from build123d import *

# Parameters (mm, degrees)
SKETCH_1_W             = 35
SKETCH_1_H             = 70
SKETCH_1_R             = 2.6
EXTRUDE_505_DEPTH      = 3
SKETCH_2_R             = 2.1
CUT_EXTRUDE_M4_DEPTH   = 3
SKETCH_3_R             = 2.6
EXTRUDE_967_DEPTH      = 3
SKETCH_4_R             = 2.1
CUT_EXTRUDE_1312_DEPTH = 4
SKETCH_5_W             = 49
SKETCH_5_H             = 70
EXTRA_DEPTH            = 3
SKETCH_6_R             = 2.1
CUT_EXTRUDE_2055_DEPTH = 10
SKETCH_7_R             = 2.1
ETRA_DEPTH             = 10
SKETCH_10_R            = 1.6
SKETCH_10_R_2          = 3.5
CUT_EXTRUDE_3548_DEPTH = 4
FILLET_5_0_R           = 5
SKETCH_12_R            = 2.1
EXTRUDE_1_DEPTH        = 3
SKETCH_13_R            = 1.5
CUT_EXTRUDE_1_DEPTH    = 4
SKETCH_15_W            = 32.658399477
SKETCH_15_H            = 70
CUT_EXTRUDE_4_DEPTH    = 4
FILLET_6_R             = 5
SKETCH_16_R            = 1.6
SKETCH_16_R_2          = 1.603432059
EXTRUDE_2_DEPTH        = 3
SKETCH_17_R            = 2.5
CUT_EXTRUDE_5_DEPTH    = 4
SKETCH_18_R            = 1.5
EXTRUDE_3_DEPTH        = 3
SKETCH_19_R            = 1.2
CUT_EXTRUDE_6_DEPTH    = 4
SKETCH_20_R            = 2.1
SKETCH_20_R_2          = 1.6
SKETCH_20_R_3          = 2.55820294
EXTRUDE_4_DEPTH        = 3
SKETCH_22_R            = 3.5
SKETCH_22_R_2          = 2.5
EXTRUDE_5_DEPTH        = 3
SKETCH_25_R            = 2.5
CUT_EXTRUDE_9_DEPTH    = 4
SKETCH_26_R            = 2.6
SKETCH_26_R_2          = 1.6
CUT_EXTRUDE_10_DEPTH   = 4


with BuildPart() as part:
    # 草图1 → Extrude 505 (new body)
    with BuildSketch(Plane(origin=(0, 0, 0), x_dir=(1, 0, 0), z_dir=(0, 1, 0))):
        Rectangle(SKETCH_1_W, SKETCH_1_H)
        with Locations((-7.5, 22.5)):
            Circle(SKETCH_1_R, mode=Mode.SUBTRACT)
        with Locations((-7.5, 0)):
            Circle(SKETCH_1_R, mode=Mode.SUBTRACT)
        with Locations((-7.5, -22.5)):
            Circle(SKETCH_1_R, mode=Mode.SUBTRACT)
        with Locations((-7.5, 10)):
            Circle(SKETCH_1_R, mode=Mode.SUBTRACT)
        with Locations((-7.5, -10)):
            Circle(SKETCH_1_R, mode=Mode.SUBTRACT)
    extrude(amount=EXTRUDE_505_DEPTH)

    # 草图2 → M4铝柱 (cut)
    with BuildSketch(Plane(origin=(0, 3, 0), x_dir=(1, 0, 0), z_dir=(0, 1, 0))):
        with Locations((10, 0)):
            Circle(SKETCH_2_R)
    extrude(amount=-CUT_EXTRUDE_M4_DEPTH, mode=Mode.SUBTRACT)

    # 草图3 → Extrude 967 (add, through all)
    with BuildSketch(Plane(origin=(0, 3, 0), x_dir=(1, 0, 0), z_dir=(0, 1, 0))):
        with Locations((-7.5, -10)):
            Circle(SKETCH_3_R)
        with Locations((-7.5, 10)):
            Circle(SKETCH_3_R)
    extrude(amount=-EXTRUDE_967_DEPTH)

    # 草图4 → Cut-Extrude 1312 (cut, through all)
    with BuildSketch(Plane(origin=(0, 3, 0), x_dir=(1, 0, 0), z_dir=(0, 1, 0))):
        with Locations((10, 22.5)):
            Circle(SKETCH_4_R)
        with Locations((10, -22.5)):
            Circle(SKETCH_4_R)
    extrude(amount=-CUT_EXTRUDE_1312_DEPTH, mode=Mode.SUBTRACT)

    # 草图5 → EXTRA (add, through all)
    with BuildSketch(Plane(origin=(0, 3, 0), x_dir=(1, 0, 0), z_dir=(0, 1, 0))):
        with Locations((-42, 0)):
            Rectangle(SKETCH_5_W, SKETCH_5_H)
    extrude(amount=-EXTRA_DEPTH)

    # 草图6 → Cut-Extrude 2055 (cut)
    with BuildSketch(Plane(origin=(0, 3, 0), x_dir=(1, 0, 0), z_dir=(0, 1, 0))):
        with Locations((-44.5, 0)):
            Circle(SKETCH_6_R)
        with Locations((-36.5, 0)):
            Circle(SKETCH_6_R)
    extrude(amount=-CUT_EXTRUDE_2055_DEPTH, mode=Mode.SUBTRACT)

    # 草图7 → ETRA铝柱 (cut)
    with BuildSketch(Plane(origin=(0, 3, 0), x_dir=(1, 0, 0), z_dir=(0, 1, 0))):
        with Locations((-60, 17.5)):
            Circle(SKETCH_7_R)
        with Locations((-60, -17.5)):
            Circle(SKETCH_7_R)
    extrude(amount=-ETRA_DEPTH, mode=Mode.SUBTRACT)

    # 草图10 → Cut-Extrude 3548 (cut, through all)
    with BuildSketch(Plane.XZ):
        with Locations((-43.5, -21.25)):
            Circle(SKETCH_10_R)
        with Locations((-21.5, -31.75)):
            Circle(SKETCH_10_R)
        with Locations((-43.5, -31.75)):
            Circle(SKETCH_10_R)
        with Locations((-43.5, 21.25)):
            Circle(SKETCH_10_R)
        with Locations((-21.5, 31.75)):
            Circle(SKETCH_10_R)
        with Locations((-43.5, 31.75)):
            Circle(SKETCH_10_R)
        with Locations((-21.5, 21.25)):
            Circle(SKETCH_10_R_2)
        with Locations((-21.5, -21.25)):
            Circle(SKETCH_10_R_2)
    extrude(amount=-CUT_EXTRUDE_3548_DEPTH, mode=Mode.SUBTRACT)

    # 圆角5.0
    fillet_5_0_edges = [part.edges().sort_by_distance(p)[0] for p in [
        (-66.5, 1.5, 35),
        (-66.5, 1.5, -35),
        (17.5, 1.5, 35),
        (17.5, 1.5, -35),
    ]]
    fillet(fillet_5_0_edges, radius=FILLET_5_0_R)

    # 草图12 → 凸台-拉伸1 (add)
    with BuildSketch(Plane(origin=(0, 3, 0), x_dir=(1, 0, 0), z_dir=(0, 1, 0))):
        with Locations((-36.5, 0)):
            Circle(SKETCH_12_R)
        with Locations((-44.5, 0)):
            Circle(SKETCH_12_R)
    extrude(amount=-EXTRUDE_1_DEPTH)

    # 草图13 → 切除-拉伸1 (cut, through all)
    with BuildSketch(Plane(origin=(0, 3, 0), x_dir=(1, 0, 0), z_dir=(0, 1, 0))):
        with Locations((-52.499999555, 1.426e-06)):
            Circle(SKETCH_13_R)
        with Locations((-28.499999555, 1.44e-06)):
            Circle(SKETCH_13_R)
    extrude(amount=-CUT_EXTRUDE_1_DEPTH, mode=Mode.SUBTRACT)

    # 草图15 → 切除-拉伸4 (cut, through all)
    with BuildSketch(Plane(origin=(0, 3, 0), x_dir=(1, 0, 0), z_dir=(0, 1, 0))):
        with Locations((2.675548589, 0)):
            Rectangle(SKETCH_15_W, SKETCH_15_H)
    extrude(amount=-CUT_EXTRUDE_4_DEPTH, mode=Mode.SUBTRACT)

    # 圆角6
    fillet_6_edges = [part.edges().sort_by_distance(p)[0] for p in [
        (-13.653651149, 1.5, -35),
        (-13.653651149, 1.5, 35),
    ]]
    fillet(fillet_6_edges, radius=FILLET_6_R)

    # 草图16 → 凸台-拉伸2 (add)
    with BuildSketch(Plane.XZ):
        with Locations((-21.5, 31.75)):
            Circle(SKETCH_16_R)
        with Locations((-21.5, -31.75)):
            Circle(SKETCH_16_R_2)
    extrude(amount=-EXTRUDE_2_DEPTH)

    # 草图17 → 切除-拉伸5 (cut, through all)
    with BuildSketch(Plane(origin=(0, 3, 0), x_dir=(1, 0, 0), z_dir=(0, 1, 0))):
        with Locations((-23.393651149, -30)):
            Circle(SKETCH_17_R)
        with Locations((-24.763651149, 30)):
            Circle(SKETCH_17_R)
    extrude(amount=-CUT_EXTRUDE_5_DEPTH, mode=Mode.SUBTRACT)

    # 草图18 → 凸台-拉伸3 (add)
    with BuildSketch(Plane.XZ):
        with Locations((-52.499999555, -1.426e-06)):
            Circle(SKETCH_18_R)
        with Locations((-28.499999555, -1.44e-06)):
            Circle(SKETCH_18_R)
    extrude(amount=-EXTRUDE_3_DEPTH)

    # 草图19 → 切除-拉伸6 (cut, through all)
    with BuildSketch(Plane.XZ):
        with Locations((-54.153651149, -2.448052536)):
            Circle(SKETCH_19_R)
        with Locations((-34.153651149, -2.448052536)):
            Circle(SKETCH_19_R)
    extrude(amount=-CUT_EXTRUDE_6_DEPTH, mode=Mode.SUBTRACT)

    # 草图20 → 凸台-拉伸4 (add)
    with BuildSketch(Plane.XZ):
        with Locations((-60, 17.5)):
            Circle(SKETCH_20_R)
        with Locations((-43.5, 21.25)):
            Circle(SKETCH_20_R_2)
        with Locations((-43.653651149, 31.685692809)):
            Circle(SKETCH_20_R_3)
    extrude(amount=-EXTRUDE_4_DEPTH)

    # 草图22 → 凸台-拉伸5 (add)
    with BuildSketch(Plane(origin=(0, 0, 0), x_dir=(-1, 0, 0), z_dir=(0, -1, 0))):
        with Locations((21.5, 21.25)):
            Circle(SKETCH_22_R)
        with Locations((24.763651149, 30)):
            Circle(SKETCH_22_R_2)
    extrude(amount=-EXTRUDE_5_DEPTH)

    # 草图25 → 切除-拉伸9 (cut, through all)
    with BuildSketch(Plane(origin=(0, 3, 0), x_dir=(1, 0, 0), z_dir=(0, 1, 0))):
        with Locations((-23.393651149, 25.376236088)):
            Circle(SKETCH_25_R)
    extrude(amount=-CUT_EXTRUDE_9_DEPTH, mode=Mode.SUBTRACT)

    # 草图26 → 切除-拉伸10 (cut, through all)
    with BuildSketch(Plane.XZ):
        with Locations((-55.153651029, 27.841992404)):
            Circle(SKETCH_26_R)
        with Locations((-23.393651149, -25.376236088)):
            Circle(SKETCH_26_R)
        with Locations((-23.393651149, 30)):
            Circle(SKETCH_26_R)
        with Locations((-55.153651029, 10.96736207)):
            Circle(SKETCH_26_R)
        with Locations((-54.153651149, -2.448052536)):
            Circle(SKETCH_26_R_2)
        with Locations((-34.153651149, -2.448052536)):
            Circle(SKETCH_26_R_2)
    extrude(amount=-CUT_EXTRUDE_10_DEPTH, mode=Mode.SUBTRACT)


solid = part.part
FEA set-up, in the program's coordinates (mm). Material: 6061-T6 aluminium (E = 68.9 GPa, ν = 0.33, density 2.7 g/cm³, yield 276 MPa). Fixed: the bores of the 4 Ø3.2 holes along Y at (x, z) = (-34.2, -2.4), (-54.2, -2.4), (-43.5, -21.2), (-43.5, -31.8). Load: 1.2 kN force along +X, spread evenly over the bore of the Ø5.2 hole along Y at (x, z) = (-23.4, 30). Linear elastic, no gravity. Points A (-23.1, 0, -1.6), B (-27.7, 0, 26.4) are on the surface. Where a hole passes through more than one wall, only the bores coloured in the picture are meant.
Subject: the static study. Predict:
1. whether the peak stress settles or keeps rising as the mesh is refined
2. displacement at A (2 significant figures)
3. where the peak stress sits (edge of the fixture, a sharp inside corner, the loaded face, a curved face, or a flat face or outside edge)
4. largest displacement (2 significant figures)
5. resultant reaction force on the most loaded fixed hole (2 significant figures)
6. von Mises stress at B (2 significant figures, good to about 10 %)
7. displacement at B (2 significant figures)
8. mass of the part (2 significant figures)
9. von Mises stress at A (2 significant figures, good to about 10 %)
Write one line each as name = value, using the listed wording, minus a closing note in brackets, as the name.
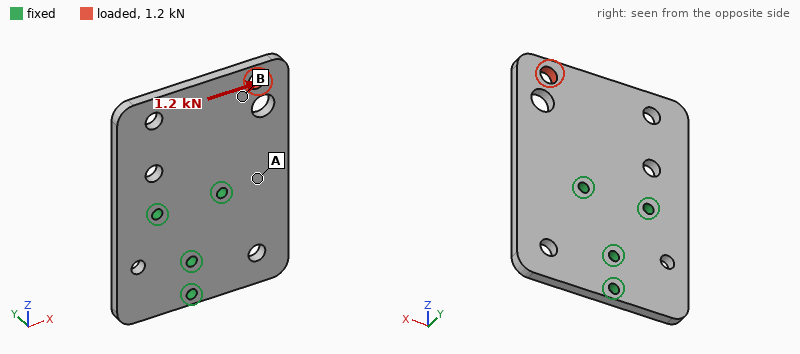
whether the peak stress settles or keeps rising as the mesh is refined = keeps rising
displacement at A = 7.9 µm
where the peak stress sits = edge of the fixture
largest displacement = 43 µm
resultant reaction force on the most loaded fixed hole = 1.4 kN
von Mises stress at B = 32 MPa
displacement at B = 29 µm
mass of the part = 28 g
von Mises stress at A = 15 MPa
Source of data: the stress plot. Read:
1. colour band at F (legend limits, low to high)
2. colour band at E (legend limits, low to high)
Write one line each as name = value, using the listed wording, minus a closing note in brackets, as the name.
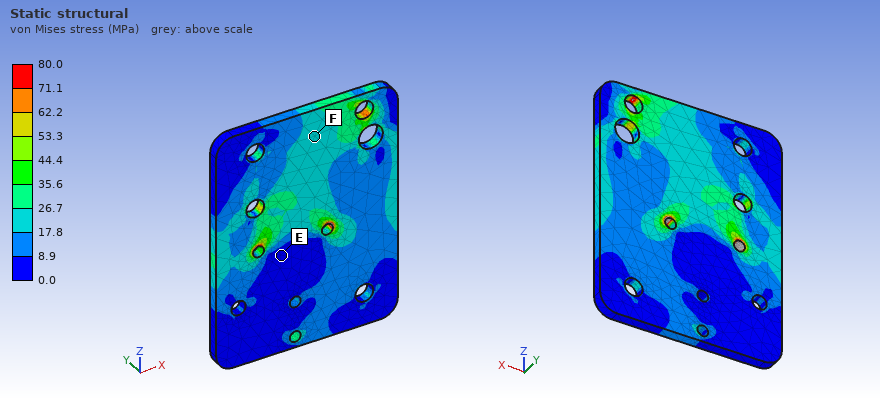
colour band at F = 17.8 to 26.7 MPa
colour band at E = 0.0 to 8.9 MPa
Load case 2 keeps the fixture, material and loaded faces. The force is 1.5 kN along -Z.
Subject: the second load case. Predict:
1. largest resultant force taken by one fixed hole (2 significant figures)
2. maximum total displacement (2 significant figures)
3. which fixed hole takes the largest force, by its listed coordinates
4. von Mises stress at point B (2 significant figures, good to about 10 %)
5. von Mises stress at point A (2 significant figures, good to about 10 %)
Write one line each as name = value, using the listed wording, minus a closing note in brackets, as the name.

largest resultant force taken by one fixed hole = 1.4 kN
maximum total displacement = 32 µm
which fixed hole takes the largest force, by its listed coordinates = (-34.2, -2.4)
von Mises stress at point B = 48 MPa
von Mises stress at point A = 16 MPa
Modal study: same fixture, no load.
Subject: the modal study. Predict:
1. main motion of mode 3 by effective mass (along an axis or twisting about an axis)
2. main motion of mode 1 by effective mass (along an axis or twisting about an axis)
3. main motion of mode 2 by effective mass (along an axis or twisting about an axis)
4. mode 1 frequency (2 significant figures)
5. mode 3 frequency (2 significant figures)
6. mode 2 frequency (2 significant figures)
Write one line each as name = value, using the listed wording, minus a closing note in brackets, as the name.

main motion of mode 3 by effective mass = along Y
main motion of mode 1 by effective mass = along Y
main motion of mode 2 by effective mass = twisting about Z
mode 1 frequency = 1700 Hz
mode 3 frequency = 4200 Hz
mode 2 frequency = 3000 Hz
